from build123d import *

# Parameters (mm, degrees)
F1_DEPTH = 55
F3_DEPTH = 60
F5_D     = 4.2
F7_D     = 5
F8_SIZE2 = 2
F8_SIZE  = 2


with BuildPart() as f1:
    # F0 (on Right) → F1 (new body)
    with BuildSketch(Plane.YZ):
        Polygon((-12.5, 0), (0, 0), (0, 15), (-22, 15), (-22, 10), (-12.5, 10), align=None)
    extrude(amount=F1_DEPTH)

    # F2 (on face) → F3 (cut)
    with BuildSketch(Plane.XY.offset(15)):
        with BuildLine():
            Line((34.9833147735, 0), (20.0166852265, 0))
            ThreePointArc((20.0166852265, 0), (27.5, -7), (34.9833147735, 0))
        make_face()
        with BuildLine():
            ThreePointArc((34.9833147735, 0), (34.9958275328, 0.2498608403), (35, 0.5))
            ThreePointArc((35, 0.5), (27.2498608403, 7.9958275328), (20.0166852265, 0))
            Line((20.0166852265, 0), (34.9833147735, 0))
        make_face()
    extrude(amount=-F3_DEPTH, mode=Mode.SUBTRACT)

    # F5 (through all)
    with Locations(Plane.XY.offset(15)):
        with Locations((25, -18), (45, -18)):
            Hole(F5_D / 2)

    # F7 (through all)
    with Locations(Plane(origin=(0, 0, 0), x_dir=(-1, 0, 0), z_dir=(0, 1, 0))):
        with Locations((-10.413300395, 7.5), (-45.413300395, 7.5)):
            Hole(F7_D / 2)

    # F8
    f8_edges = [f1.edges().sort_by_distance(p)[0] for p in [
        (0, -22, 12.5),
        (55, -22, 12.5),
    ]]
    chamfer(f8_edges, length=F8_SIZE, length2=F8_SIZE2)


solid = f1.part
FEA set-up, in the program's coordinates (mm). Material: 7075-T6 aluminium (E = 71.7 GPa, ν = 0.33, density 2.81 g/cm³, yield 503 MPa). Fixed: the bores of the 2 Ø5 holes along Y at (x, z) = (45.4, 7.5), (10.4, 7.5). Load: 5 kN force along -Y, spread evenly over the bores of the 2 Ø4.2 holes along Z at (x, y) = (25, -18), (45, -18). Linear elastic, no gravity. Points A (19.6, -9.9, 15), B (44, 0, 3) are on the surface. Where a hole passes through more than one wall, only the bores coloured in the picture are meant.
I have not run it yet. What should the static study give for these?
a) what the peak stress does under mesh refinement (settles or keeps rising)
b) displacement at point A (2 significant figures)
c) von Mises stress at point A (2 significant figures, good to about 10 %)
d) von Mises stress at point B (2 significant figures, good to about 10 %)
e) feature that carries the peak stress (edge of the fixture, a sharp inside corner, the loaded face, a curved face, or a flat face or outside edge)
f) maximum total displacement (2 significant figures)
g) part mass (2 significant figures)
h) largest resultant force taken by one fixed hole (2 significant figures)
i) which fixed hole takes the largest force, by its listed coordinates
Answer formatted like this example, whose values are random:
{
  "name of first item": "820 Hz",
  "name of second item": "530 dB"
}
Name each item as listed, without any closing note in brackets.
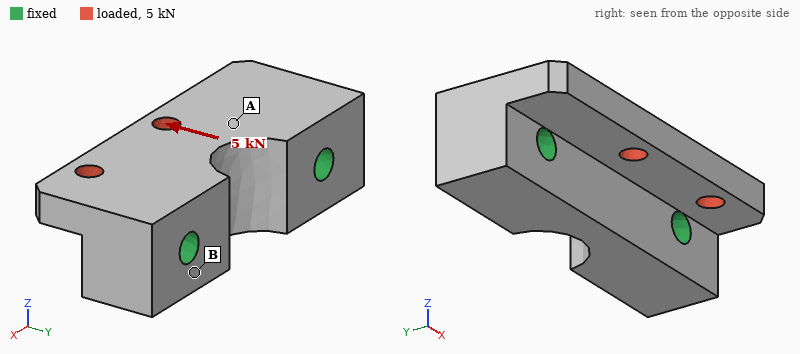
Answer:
{
  "what the peak stress does under mesh refinement": "keeps rising",
  "displacement at point A": "8.2 µm",
  "von Mises stress at point A": "40 MPa",
  "von Mises stress at point B": "17 MPa",
  "feature that carries the peak stress": "edge of the fixture",
  "maximum total displacement": "22 µm",
  "part mass": "31 g",
  "largest resultant force taken by one fixed hole": "3.5 kN",
  "which fixed hole takes the largest force, by its listed coordinates": "(45.4, 7.5)"
}
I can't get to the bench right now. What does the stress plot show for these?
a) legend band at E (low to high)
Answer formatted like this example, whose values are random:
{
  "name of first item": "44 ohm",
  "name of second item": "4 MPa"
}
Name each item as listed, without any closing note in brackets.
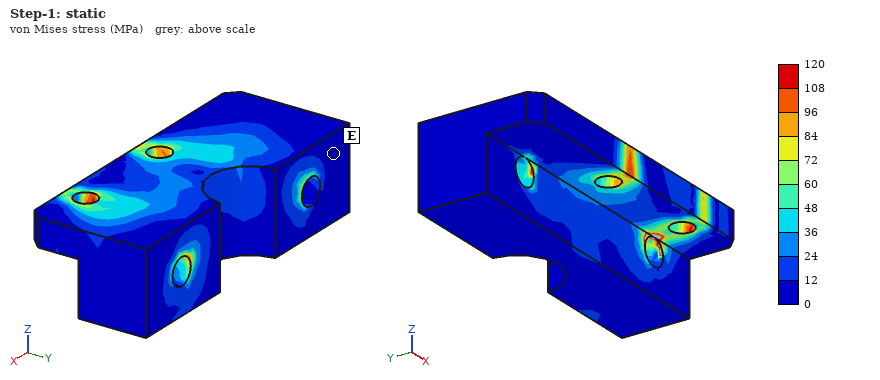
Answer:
{
  "legend band at E": "0 to 12 MPa"
}
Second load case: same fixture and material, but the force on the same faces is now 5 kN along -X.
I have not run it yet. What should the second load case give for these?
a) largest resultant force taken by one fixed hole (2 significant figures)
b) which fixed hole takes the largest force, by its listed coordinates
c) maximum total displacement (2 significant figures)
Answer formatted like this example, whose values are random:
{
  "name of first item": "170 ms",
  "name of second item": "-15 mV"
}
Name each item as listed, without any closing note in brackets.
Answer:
{
  "largest resultant force taken by one fixed hole": "3.1 kN",
  "which fixed hole takes the largest force, by its listed coordinates": "(45.4, 7.5)",
  "maximum total displacement": "18 µm"
}
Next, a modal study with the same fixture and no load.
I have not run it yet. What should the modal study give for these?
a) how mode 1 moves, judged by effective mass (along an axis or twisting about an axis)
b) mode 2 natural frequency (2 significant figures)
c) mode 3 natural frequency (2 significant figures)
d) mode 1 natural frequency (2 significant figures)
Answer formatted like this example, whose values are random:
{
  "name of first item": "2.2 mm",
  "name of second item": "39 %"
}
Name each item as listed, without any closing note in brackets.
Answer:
{
  "how mode 1 moves, judged by effective mass": "along Z",
  "mode 2 natural frequency": "27 kHz",
  "mode 3 natural frequency": "29 kHz",
  "mode 1 natural frequency": "21 kHz"
}
